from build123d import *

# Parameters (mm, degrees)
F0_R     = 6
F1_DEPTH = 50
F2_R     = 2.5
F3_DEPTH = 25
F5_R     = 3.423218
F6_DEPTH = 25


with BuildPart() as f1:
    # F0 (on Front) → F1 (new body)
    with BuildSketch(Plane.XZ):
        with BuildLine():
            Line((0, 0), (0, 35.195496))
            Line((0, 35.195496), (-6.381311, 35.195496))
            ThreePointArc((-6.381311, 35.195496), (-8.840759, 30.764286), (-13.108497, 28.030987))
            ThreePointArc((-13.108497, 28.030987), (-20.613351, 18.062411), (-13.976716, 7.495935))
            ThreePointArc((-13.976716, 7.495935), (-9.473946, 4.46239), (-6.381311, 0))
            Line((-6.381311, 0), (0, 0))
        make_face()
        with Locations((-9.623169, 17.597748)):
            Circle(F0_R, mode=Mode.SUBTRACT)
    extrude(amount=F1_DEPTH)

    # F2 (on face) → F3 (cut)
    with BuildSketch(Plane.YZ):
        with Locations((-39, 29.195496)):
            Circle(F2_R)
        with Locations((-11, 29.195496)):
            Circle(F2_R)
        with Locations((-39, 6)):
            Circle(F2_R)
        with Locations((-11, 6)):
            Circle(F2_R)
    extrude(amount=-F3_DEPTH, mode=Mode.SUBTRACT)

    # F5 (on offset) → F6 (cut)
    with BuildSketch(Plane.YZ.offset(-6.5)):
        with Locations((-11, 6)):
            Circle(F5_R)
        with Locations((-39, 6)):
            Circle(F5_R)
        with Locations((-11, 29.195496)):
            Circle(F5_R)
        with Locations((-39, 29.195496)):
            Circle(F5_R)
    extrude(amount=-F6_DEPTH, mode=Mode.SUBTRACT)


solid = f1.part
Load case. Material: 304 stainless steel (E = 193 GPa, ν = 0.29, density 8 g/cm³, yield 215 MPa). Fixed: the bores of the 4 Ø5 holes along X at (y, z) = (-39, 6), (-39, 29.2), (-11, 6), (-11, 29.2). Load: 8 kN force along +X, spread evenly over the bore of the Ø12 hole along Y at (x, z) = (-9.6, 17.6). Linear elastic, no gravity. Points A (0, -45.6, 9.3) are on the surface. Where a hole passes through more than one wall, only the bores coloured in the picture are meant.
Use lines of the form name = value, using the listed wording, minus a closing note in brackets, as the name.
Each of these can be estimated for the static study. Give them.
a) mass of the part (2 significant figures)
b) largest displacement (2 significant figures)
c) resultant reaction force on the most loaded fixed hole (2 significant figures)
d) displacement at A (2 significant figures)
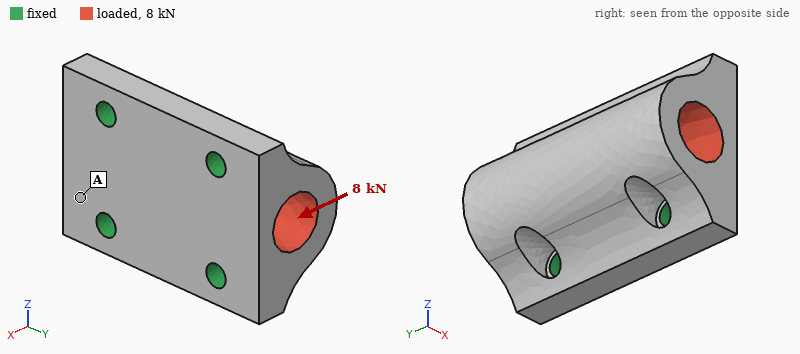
mass of the part = 150 g
largest displacement = 2.5 µm
resultant reaction force on the most loaded fixed hole = 2.0 kN
displacement at A = 1.2 µm
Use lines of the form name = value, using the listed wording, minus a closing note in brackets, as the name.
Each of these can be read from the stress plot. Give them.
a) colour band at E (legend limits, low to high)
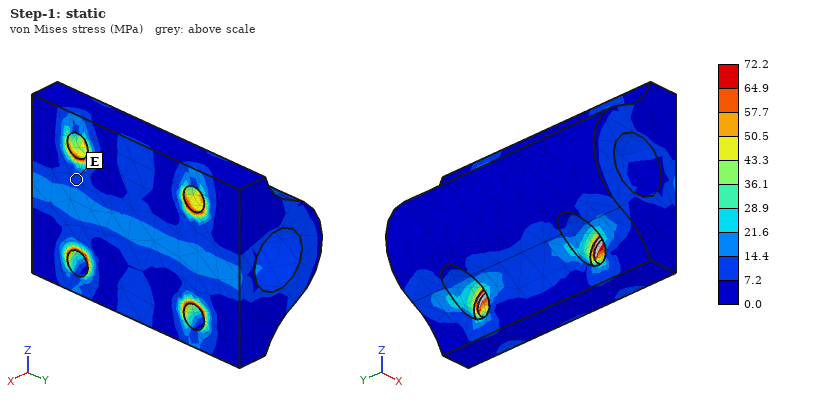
colour band at E = 7.2 to 14.4 MPa
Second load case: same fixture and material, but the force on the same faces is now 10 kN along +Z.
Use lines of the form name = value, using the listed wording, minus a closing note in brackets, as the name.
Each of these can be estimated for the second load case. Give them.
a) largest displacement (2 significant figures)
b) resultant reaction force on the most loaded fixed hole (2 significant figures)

largest displacement = 4.4 µm
resultant reaction force on the most loaded fixed hole = 2.7 kN
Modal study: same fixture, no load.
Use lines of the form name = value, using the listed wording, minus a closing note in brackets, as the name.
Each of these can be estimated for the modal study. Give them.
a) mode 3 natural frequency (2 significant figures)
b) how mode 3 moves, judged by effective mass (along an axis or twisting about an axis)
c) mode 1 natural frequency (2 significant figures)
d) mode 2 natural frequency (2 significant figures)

mode 3 natural frequency = 31 kHz
how mode 3 moves, judged by effective mass = twisting about X
mode 1 natural frequency = 25 kHz
mode 2 natural frequency = 26 kHz
